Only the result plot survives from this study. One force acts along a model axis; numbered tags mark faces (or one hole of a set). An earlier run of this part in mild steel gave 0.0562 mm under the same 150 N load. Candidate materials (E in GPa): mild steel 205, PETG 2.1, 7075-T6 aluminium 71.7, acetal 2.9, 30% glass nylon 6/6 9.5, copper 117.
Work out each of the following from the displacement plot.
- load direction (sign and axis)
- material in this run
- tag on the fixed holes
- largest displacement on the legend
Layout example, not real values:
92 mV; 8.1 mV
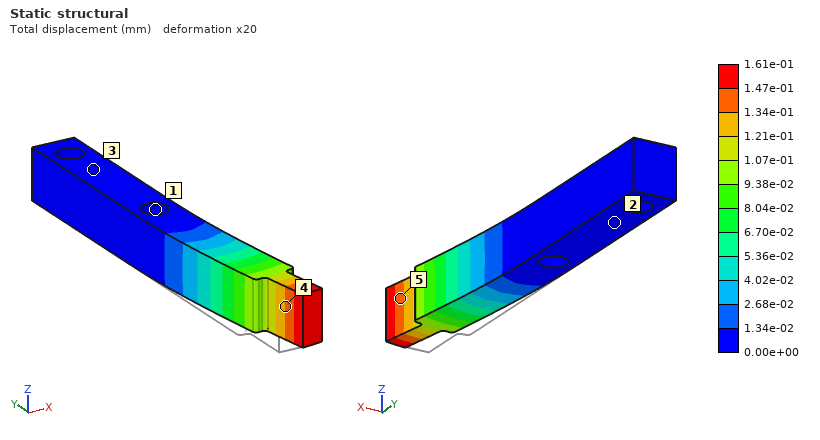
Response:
+X; 7075-T6 aluminium; 1; 1.61e-01 mm
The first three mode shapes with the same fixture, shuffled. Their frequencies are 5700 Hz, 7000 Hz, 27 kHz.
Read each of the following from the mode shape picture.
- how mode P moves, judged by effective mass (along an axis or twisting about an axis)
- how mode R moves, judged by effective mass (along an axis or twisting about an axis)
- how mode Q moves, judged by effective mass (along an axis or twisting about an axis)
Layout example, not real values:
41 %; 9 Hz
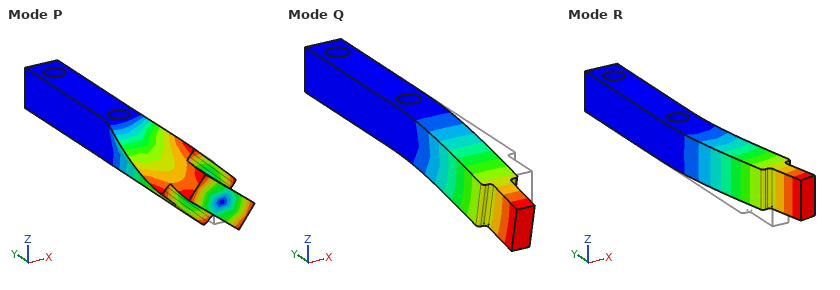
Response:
twisting about Y; along X; along Z
